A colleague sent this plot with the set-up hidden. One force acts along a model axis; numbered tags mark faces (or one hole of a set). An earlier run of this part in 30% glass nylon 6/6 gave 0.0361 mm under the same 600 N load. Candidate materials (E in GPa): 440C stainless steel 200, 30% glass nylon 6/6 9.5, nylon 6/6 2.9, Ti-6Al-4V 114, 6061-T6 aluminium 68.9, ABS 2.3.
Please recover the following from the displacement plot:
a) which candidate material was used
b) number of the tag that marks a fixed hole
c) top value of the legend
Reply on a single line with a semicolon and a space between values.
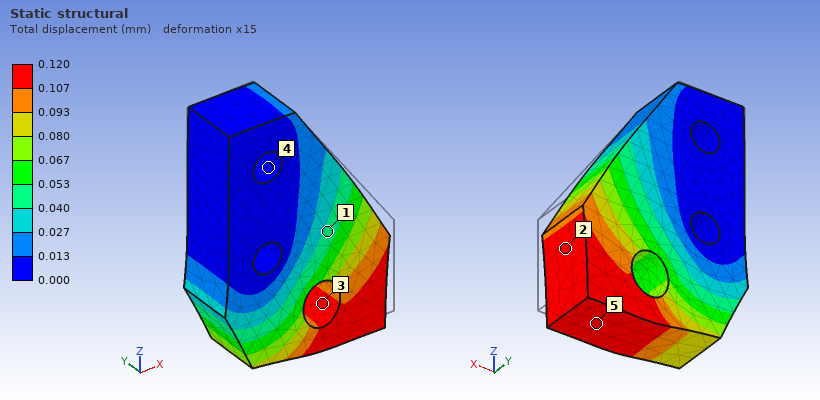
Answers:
nylon 6/6; 4; 0.120 mm
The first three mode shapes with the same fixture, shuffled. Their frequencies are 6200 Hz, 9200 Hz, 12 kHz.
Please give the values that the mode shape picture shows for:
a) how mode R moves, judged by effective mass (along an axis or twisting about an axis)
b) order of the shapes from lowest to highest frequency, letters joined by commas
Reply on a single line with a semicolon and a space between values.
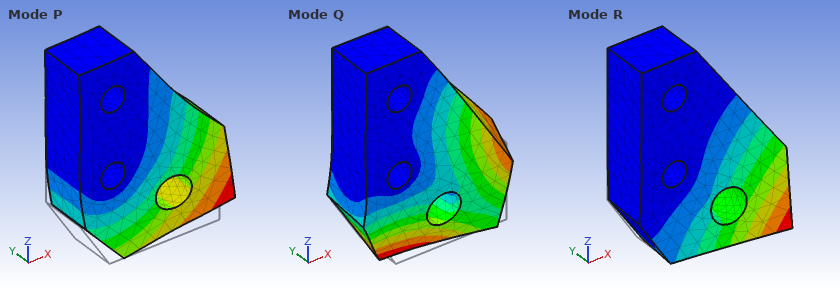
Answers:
along Y; R, P, Q
